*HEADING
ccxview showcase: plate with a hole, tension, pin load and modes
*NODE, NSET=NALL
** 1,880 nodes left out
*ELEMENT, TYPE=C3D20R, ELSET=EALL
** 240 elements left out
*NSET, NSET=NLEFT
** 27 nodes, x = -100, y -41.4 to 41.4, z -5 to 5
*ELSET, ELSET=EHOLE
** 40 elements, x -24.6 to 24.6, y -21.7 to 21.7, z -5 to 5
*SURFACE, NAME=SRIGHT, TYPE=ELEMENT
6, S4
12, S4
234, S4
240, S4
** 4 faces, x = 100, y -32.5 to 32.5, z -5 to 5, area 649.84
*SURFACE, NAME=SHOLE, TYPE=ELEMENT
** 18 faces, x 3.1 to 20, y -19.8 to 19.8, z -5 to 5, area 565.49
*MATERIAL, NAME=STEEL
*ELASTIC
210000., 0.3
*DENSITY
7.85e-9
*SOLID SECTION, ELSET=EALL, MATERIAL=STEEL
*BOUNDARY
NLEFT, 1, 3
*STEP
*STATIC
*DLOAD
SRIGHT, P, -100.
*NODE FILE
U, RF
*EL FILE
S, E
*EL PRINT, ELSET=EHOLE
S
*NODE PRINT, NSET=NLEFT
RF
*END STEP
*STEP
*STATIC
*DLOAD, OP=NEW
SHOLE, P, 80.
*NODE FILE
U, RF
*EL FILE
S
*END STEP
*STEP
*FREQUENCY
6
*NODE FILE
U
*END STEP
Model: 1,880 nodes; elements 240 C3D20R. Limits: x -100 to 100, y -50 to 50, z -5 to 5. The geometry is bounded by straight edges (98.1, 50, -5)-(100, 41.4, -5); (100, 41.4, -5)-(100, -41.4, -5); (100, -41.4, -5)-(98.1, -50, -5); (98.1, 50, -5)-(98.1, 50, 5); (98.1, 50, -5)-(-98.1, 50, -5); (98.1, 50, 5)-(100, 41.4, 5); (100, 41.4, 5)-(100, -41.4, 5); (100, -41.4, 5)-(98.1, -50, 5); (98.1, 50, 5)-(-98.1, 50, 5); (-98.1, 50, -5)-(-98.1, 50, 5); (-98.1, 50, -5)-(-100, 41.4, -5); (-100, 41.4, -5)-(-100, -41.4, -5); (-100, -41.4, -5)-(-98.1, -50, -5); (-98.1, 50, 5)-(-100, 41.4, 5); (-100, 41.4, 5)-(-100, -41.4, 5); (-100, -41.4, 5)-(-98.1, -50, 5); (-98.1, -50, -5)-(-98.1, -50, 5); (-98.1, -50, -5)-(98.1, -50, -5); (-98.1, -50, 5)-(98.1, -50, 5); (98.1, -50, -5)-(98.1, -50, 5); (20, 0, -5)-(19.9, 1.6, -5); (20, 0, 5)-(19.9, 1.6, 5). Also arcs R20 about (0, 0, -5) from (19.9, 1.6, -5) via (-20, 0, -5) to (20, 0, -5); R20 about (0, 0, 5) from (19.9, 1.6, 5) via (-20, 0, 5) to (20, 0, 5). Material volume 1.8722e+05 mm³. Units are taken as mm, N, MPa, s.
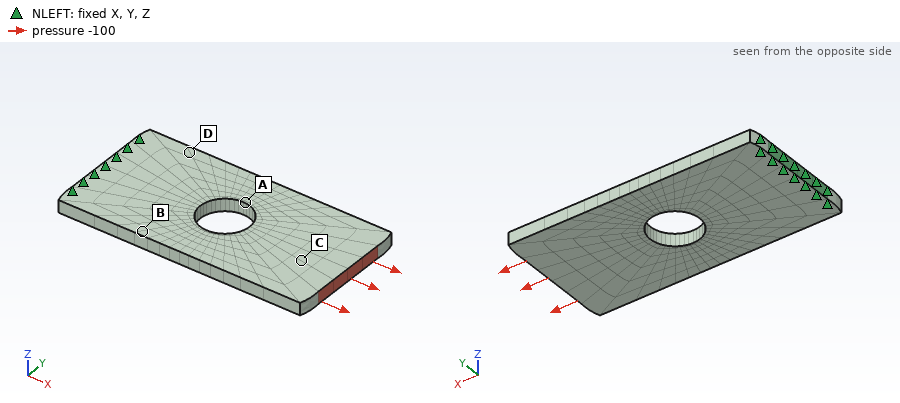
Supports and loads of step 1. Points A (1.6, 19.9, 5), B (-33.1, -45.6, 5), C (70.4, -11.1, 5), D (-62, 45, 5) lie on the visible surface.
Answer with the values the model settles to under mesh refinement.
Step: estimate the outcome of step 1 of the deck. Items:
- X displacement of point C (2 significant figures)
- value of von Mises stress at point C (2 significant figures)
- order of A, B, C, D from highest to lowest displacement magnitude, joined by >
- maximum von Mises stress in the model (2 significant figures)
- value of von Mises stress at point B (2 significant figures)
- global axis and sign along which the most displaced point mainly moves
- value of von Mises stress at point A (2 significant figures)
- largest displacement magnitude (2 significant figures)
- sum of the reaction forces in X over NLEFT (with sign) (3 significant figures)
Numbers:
0.074 mm
85 MPa
C > A > B > D
250 MPa
92 MPa
+X
250 MPa
0.087 mm
-65000 N
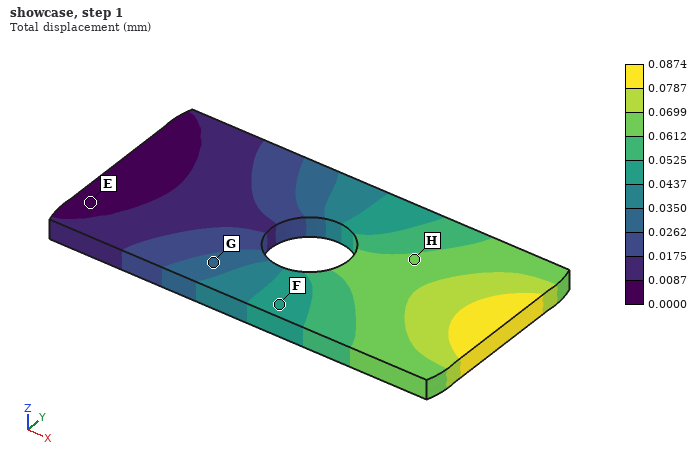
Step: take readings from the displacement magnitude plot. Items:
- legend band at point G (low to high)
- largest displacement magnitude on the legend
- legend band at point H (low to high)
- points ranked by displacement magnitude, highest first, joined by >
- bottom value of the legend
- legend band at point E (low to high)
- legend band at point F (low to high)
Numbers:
0.0262 to 0.0350 mm
0.0874 mm
0.0612 to 0.0699 mm
H > F > G > E
0.0000 mm
0.0000 to 0.0087 mm
0.0437 to 0.0525 mm
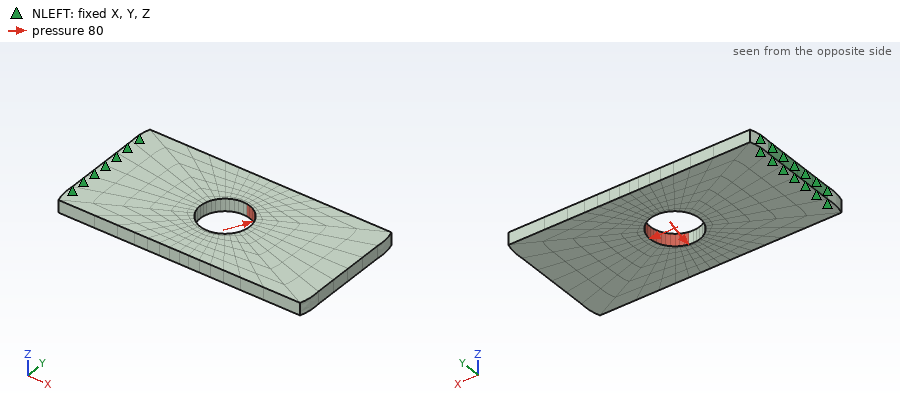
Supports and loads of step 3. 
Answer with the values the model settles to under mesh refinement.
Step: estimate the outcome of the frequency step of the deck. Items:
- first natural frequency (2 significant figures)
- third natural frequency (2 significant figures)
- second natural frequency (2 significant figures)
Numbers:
210 Hz
1200 Hz
820 Hz
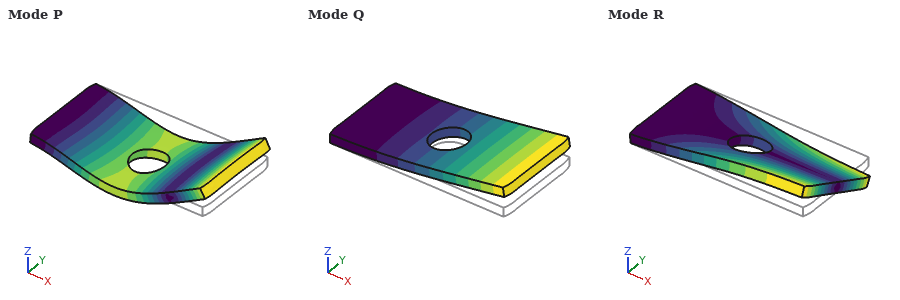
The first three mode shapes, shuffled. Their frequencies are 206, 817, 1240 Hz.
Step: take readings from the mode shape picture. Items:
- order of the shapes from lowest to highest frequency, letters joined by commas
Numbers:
Q, R, P
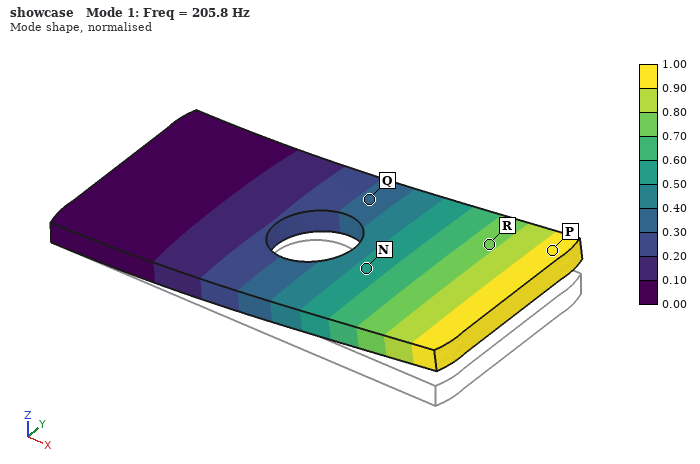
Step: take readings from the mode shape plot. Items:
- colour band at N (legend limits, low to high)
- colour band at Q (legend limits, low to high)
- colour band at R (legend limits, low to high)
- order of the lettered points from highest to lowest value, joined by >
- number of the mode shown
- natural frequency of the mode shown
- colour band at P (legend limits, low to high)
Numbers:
0.50 to 0.60
0.30 to 0.40
0.70 to 0.80
P > R > N > Q
1
205.8 Hz
0.90 to 1.00
